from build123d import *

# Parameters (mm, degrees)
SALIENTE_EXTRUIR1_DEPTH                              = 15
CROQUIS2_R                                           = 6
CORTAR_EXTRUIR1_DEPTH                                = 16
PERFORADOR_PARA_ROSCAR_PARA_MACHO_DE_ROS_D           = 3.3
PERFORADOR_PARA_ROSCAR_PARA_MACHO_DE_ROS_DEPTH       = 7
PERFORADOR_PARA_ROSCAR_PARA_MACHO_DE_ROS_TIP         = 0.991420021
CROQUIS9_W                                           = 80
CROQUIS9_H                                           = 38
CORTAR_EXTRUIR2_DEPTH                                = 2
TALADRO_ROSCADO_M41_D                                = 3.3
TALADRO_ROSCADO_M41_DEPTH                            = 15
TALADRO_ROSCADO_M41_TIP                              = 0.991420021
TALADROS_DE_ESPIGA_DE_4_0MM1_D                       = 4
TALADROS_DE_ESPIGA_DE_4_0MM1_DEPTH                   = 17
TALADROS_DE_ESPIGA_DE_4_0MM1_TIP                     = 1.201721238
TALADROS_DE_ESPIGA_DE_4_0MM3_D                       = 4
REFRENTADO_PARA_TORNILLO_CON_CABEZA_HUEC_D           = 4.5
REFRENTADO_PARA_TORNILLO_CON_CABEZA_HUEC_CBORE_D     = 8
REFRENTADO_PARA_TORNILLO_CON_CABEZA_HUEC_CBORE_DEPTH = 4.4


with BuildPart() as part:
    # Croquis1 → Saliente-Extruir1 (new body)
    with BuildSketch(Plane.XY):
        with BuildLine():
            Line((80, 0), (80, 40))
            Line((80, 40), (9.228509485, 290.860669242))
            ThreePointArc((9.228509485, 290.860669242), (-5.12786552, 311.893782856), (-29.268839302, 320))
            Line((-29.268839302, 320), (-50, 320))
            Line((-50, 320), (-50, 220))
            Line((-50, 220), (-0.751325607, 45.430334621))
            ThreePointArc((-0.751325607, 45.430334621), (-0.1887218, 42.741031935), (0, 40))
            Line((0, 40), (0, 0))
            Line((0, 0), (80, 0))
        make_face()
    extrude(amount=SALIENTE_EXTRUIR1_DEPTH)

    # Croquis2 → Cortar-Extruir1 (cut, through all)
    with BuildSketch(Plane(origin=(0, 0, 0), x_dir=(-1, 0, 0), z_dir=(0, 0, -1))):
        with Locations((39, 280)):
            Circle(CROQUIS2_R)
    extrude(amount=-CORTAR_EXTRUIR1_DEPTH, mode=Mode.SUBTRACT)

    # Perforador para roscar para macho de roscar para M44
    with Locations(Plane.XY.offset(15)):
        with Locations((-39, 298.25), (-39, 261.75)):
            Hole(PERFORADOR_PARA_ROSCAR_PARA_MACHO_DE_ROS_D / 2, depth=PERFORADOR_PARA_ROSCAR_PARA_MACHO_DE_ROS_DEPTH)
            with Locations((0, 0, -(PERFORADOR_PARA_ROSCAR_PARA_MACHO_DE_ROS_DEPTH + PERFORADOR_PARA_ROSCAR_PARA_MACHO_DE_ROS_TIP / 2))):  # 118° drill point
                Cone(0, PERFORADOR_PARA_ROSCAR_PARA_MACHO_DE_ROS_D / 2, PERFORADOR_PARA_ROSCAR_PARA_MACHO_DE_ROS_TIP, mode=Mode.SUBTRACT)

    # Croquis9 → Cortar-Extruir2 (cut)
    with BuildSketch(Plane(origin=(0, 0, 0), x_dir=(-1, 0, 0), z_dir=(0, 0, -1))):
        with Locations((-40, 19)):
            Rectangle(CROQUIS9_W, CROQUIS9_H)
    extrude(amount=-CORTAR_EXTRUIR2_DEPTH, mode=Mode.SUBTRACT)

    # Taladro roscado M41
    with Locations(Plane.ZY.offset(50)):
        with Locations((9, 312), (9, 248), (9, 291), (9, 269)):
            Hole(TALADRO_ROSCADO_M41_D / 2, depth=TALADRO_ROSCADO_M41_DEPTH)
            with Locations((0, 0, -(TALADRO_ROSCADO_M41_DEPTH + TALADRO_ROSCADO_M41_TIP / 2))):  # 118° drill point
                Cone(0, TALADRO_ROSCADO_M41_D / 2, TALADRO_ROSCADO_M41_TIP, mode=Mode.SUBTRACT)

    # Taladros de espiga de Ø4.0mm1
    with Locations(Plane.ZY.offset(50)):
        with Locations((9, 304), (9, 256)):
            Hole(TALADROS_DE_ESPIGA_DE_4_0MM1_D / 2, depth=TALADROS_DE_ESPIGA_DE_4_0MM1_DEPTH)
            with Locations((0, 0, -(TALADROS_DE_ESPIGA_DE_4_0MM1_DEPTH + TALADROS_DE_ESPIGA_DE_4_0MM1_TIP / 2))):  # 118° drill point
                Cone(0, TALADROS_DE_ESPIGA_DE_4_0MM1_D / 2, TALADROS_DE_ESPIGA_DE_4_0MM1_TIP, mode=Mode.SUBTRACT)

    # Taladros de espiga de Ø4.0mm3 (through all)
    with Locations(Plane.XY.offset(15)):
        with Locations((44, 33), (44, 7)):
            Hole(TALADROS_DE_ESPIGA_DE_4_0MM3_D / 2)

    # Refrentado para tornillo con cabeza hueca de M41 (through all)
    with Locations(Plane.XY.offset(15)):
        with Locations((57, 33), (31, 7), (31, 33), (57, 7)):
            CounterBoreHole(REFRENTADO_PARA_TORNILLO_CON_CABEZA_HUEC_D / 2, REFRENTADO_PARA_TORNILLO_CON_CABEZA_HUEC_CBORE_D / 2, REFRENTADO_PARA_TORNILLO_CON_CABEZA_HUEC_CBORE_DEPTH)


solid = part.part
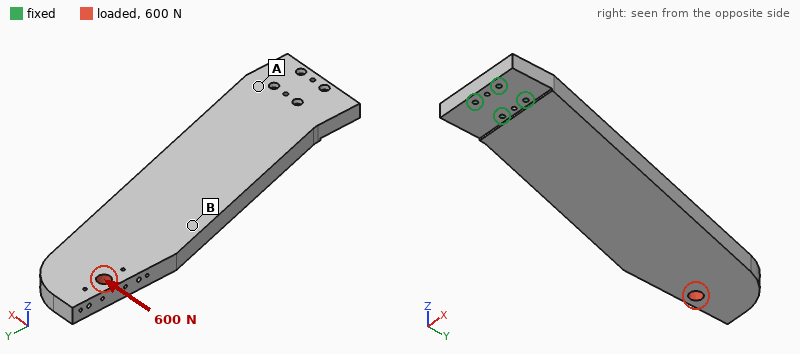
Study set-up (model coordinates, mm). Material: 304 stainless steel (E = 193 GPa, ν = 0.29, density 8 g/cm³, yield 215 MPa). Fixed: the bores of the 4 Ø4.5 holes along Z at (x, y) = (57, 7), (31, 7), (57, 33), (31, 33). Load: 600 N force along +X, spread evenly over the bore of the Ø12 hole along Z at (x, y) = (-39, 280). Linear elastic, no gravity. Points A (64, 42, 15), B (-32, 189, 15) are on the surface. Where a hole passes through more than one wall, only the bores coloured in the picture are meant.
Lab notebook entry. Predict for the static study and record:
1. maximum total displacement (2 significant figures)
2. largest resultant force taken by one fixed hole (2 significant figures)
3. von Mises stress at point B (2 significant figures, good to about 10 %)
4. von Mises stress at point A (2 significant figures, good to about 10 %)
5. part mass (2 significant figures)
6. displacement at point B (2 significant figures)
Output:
56 µm
2.8 kN
2.5 MPa
6.9 MPa
2.8 kg
27 µm
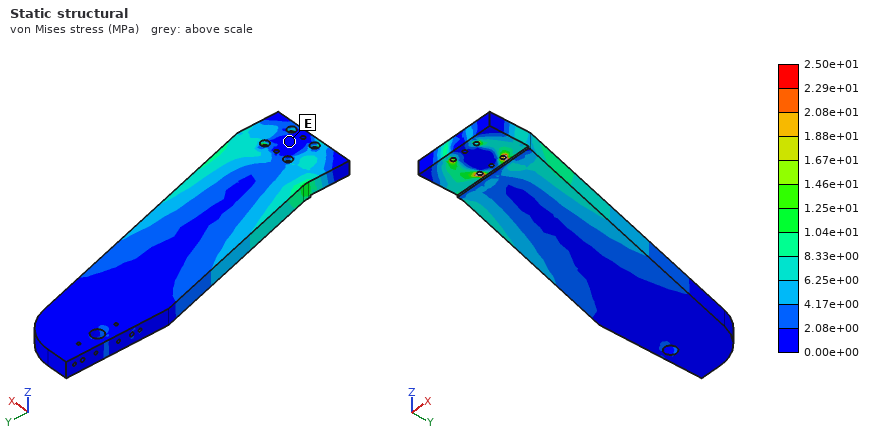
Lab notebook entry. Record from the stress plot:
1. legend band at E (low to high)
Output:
0.00e+00 to 2.08e+00 MPa
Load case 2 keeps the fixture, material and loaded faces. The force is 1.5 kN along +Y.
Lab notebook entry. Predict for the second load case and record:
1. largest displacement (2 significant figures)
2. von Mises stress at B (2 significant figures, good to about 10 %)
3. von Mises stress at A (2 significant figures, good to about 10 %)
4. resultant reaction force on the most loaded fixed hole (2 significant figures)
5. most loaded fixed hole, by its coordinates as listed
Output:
50 µm
4.0 MPa
4.5 MPa
2.6 kN
(31, 33)
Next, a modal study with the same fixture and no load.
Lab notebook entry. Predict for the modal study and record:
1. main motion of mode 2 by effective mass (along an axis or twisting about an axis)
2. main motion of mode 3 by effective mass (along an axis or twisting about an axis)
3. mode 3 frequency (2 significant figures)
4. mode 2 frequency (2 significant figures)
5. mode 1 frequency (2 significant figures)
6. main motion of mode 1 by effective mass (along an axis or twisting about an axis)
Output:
along X
along Z
830 Hz
600 Hz
140 Hz
along Z
